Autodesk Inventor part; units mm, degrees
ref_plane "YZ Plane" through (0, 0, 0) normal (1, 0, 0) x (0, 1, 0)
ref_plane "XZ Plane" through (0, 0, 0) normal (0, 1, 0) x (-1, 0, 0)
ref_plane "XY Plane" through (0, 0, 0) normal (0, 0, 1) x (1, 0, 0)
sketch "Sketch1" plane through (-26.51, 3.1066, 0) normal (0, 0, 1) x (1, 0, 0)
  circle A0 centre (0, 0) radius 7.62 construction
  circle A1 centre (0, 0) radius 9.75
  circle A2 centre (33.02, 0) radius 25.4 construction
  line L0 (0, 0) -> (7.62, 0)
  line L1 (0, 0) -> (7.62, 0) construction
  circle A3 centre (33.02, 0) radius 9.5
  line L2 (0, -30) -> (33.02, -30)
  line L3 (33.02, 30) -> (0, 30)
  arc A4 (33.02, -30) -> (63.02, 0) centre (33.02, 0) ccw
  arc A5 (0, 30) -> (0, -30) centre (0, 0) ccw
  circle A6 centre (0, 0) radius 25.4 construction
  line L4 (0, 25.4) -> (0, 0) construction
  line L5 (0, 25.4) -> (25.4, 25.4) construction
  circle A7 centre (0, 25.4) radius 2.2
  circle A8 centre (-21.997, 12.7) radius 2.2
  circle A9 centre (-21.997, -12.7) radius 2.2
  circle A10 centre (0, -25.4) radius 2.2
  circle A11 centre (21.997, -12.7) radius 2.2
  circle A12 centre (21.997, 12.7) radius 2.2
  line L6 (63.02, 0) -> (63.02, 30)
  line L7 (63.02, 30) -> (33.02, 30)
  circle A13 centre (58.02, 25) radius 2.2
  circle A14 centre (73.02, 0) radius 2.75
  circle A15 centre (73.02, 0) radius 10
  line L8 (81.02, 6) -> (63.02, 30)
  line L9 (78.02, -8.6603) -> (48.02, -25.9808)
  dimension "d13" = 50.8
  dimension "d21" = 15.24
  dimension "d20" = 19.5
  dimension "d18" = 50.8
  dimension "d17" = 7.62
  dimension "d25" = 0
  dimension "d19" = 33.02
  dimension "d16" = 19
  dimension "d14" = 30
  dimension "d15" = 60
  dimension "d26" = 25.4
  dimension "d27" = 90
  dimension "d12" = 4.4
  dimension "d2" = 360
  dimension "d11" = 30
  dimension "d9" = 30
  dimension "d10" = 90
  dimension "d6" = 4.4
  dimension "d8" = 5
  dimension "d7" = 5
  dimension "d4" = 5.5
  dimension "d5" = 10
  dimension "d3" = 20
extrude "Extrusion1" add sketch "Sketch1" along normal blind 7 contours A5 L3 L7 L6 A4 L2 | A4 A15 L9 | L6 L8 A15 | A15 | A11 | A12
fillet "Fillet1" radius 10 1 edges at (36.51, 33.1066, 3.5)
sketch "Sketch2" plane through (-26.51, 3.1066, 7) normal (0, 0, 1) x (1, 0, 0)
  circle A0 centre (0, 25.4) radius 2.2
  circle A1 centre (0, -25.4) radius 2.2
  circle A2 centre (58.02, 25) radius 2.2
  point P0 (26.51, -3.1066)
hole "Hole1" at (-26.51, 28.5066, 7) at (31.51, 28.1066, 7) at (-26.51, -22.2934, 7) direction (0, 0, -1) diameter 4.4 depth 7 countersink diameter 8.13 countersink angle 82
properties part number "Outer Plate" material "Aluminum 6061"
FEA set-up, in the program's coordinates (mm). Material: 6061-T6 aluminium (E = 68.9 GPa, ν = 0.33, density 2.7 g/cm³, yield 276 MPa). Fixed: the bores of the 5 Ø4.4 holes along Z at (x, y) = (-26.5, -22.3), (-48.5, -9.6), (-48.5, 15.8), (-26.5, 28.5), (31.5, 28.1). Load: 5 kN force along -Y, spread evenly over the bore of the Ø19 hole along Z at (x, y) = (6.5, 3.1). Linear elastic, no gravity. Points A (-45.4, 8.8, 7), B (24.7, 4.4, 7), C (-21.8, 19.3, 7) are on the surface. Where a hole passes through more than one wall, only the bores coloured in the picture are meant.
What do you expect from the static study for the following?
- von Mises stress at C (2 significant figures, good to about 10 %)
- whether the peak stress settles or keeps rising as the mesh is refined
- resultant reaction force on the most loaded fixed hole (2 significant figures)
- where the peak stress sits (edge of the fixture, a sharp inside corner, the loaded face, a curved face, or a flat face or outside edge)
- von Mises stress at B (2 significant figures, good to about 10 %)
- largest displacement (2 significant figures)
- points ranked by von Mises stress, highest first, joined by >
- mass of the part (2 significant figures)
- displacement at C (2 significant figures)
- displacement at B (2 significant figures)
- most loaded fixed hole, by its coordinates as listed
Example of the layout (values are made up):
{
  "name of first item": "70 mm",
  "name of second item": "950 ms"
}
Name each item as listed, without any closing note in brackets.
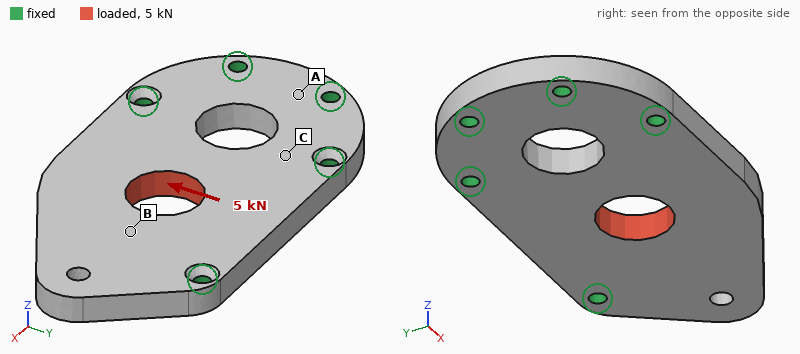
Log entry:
{
  "von Mises stress at C": "17 MPa",
  "whether the peak stress settles or keeps rising as the mesh is refined": "keeps rising",
  "resultant reaction force on the most loaded fixed hole": "2.6 kN",
  "where the peak stress sits": "edge of the fixture",
  "von Mises stress at B": "11 MPa",
  "largest displacement": "13 µm",
  "points ranked by von Mises stress, highest first, joined by >": "C > B > A",
  "mass of the part": "93 g",
  "displacement at C": "3.6 µm",
  "displacement at B": "8.9 µm",
  "most loaded fixed hole, by its coordinates as listed": "(31.5, 28.1)"
}
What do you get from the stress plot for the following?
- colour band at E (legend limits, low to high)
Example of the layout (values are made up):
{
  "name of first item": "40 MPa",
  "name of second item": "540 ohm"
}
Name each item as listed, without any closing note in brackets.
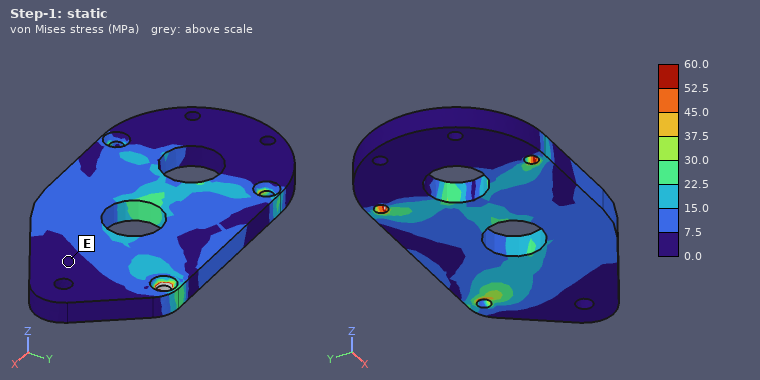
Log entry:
{
  "colour band at E": "0.0 to 7.5 MPa"
}
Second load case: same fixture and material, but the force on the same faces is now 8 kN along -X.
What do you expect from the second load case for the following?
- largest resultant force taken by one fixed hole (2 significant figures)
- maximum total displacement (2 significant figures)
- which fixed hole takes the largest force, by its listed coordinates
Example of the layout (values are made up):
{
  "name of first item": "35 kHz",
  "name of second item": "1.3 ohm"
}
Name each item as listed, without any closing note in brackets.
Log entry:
{
  "largest resultant force taken by one fixed hole": "2.6 kN",
  "maximum total displacement": "17 µm",
  "which fixed hole takes the largest force, by its listed coordinates": "(-26.5, -22.3)"
}
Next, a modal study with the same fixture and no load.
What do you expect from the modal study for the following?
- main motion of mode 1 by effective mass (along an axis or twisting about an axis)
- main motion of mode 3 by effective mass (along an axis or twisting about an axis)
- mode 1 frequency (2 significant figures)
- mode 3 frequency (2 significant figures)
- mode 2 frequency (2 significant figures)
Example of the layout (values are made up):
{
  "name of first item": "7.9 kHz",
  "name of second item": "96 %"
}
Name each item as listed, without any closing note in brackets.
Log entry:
{
  "main motion of mode 1 by effective mass": "along Z",
  "main motion of mode 3 by effective mass": "along Z",
  "mode 1 frequency": "2800 Hz",
  "mode 3 frequency": "8700 Hz",
  "mode 2 frequency": "5800 Hz"
}
